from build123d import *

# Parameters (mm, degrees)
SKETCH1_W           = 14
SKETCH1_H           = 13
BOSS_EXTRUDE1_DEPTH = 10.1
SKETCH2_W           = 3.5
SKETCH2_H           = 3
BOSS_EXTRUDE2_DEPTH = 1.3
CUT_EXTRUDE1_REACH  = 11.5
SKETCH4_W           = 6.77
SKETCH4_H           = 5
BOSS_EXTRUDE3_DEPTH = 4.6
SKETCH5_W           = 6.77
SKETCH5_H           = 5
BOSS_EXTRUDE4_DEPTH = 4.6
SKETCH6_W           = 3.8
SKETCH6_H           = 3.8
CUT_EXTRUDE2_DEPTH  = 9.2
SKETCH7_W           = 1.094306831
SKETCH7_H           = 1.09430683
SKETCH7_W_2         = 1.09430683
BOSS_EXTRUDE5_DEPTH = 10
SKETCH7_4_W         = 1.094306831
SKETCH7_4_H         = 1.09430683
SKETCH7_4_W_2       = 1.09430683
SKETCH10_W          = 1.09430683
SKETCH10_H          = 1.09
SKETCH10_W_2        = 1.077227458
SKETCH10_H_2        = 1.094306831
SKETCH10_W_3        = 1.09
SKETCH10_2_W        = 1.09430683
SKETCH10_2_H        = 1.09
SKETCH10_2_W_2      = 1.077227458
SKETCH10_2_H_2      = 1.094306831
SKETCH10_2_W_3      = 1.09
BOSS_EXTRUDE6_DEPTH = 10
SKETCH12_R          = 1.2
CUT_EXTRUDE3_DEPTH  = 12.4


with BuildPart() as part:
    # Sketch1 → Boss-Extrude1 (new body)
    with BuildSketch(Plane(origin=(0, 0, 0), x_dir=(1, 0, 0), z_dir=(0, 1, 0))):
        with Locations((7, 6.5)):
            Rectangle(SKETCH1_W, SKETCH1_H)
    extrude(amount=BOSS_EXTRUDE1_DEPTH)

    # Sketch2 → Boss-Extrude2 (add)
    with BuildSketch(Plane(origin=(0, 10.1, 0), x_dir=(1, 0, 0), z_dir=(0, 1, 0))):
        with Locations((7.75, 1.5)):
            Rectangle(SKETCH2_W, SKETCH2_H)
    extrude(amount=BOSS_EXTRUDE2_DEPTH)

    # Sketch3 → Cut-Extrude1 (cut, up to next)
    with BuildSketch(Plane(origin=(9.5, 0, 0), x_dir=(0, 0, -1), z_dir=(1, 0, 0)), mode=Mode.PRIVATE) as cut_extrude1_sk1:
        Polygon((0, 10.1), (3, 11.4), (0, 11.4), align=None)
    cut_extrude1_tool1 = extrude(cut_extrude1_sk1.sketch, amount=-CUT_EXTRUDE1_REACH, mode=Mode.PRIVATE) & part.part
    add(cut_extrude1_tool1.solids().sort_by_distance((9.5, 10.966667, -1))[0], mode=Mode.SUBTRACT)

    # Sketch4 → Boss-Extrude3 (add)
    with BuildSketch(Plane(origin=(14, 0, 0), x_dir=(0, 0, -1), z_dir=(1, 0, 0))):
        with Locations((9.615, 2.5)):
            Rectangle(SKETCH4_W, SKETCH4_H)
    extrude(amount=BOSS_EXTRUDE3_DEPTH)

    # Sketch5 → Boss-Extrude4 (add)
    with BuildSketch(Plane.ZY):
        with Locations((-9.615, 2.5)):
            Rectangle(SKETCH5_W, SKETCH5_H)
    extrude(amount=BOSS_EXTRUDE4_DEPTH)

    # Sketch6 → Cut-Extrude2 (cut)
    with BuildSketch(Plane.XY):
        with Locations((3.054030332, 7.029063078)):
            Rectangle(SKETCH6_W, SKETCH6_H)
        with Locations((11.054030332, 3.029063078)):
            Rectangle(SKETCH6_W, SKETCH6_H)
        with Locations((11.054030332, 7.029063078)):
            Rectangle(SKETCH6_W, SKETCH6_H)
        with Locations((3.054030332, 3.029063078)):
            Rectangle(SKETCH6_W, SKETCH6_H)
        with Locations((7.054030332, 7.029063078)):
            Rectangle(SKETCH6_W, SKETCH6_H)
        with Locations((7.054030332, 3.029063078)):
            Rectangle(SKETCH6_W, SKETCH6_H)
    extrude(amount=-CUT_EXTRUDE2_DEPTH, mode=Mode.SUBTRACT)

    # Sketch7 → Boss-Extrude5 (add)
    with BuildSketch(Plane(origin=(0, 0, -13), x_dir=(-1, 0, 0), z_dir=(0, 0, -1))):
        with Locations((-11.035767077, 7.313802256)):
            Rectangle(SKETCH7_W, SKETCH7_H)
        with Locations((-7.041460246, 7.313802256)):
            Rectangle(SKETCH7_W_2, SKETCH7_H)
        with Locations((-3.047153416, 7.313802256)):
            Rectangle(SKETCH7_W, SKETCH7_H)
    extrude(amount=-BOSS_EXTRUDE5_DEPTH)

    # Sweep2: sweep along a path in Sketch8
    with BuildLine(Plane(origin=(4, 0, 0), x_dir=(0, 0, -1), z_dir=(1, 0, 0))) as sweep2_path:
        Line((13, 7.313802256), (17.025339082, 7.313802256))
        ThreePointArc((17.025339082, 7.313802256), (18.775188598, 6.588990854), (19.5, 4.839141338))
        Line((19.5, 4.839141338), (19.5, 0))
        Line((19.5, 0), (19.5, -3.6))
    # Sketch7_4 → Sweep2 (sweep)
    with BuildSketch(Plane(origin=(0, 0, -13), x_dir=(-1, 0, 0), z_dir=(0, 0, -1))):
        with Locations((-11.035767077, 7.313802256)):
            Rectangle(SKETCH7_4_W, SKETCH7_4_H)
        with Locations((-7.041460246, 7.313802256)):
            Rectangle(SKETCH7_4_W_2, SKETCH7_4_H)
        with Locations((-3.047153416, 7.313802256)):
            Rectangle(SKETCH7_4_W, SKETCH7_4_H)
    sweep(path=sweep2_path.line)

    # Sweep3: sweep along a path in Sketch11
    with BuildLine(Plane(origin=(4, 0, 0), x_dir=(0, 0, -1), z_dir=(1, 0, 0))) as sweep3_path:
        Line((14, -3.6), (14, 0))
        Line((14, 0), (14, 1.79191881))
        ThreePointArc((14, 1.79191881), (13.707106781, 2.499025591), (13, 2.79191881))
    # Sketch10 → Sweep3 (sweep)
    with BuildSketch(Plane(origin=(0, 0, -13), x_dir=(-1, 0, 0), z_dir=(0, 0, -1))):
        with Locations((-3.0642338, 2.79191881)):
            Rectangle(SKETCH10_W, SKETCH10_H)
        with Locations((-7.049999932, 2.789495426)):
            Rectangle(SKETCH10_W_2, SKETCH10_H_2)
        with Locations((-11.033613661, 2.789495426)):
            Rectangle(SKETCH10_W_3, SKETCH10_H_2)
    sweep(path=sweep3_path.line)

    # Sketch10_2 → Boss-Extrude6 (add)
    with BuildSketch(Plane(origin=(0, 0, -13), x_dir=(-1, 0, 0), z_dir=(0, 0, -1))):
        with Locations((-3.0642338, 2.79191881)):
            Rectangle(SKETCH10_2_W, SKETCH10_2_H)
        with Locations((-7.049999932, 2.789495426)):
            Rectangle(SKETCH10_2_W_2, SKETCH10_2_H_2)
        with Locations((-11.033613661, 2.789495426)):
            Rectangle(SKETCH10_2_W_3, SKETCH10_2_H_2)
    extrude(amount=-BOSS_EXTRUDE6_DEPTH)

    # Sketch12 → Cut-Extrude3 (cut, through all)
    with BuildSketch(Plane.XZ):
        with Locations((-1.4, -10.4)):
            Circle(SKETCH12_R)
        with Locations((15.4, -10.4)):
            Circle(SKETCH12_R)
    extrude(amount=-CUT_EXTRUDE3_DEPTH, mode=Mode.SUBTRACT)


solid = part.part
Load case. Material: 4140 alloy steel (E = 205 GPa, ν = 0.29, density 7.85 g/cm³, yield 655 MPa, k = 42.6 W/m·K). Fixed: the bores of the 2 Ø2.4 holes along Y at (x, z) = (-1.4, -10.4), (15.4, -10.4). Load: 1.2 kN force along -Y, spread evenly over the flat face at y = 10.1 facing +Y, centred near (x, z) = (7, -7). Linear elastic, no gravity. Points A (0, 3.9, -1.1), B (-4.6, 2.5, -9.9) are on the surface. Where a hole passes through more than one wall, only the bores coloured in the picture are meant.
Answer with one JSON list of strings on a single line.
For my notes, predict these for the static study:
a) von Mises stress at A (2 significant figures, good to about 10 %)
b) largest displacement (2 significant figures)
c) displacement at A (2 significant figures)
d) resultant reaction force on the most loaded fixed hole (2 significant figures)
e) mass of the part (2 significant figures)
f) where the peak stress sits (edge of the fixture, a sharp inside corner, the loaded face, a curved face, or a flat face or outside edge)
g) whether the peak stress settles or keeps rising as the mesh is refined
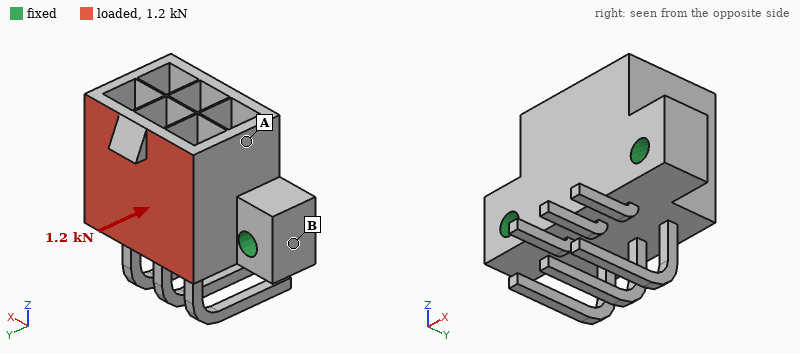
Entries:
["27 MPa", "13 µm", "6.3 µm", "630 N", "11 g", "edge of the fixture", "keeps rising"]
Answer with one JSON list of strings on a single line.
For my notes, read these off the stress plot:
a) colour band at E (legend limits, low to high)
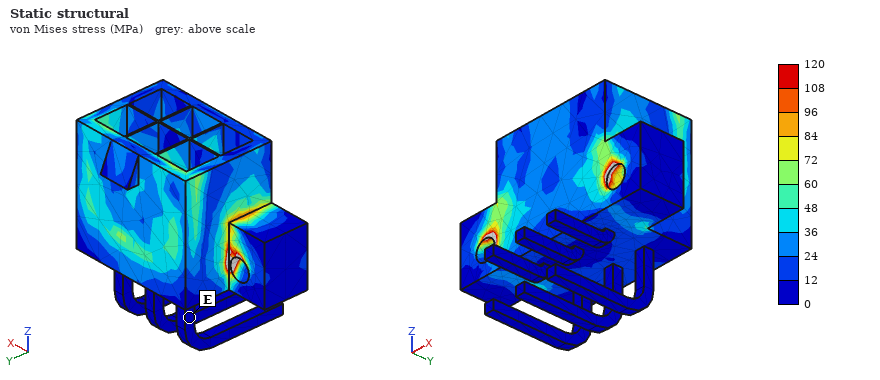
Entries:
["0 to 12 MPa"]
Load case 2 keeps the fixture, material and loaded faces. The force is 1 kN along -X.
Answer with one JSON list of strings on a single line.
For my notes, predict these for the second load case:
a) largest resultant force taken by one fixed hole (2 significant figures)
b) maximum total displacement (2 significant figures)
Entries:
["720 N", "11 µm"]
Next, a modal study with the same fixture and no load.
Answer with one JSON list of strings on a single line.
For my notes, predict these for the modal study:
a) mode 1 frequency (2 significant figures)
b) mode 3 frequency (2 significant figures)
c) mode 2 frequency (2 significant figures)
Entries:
["3500 Hz", "3500 Hz", "3500 Hz"]
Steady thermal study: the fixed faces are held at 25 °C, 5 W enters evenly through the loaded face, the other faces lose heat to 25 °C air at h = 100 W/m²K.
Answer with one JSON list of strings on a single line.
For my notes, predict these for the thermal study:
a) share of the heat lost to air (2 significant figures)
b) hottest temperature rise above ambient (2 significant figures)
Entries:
["26 %", "18 K"]
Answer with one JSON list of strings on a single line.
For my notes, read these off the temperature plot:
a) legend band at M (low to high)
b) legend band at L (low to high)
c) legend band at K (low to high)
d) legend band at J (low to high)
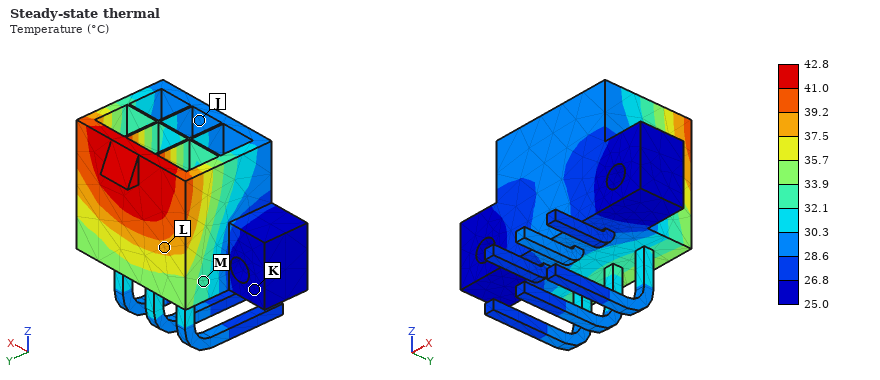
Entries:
["32.1 to 33.9 °C", "37.5 to 39.2 °C", "25.0 to 26.8 °C", "28.6 to 30.3 °C"]
